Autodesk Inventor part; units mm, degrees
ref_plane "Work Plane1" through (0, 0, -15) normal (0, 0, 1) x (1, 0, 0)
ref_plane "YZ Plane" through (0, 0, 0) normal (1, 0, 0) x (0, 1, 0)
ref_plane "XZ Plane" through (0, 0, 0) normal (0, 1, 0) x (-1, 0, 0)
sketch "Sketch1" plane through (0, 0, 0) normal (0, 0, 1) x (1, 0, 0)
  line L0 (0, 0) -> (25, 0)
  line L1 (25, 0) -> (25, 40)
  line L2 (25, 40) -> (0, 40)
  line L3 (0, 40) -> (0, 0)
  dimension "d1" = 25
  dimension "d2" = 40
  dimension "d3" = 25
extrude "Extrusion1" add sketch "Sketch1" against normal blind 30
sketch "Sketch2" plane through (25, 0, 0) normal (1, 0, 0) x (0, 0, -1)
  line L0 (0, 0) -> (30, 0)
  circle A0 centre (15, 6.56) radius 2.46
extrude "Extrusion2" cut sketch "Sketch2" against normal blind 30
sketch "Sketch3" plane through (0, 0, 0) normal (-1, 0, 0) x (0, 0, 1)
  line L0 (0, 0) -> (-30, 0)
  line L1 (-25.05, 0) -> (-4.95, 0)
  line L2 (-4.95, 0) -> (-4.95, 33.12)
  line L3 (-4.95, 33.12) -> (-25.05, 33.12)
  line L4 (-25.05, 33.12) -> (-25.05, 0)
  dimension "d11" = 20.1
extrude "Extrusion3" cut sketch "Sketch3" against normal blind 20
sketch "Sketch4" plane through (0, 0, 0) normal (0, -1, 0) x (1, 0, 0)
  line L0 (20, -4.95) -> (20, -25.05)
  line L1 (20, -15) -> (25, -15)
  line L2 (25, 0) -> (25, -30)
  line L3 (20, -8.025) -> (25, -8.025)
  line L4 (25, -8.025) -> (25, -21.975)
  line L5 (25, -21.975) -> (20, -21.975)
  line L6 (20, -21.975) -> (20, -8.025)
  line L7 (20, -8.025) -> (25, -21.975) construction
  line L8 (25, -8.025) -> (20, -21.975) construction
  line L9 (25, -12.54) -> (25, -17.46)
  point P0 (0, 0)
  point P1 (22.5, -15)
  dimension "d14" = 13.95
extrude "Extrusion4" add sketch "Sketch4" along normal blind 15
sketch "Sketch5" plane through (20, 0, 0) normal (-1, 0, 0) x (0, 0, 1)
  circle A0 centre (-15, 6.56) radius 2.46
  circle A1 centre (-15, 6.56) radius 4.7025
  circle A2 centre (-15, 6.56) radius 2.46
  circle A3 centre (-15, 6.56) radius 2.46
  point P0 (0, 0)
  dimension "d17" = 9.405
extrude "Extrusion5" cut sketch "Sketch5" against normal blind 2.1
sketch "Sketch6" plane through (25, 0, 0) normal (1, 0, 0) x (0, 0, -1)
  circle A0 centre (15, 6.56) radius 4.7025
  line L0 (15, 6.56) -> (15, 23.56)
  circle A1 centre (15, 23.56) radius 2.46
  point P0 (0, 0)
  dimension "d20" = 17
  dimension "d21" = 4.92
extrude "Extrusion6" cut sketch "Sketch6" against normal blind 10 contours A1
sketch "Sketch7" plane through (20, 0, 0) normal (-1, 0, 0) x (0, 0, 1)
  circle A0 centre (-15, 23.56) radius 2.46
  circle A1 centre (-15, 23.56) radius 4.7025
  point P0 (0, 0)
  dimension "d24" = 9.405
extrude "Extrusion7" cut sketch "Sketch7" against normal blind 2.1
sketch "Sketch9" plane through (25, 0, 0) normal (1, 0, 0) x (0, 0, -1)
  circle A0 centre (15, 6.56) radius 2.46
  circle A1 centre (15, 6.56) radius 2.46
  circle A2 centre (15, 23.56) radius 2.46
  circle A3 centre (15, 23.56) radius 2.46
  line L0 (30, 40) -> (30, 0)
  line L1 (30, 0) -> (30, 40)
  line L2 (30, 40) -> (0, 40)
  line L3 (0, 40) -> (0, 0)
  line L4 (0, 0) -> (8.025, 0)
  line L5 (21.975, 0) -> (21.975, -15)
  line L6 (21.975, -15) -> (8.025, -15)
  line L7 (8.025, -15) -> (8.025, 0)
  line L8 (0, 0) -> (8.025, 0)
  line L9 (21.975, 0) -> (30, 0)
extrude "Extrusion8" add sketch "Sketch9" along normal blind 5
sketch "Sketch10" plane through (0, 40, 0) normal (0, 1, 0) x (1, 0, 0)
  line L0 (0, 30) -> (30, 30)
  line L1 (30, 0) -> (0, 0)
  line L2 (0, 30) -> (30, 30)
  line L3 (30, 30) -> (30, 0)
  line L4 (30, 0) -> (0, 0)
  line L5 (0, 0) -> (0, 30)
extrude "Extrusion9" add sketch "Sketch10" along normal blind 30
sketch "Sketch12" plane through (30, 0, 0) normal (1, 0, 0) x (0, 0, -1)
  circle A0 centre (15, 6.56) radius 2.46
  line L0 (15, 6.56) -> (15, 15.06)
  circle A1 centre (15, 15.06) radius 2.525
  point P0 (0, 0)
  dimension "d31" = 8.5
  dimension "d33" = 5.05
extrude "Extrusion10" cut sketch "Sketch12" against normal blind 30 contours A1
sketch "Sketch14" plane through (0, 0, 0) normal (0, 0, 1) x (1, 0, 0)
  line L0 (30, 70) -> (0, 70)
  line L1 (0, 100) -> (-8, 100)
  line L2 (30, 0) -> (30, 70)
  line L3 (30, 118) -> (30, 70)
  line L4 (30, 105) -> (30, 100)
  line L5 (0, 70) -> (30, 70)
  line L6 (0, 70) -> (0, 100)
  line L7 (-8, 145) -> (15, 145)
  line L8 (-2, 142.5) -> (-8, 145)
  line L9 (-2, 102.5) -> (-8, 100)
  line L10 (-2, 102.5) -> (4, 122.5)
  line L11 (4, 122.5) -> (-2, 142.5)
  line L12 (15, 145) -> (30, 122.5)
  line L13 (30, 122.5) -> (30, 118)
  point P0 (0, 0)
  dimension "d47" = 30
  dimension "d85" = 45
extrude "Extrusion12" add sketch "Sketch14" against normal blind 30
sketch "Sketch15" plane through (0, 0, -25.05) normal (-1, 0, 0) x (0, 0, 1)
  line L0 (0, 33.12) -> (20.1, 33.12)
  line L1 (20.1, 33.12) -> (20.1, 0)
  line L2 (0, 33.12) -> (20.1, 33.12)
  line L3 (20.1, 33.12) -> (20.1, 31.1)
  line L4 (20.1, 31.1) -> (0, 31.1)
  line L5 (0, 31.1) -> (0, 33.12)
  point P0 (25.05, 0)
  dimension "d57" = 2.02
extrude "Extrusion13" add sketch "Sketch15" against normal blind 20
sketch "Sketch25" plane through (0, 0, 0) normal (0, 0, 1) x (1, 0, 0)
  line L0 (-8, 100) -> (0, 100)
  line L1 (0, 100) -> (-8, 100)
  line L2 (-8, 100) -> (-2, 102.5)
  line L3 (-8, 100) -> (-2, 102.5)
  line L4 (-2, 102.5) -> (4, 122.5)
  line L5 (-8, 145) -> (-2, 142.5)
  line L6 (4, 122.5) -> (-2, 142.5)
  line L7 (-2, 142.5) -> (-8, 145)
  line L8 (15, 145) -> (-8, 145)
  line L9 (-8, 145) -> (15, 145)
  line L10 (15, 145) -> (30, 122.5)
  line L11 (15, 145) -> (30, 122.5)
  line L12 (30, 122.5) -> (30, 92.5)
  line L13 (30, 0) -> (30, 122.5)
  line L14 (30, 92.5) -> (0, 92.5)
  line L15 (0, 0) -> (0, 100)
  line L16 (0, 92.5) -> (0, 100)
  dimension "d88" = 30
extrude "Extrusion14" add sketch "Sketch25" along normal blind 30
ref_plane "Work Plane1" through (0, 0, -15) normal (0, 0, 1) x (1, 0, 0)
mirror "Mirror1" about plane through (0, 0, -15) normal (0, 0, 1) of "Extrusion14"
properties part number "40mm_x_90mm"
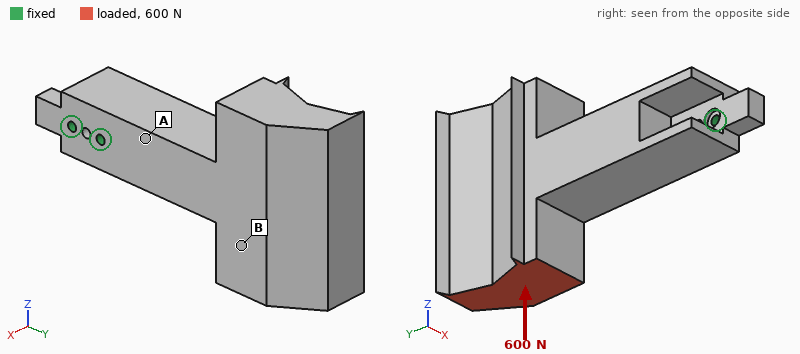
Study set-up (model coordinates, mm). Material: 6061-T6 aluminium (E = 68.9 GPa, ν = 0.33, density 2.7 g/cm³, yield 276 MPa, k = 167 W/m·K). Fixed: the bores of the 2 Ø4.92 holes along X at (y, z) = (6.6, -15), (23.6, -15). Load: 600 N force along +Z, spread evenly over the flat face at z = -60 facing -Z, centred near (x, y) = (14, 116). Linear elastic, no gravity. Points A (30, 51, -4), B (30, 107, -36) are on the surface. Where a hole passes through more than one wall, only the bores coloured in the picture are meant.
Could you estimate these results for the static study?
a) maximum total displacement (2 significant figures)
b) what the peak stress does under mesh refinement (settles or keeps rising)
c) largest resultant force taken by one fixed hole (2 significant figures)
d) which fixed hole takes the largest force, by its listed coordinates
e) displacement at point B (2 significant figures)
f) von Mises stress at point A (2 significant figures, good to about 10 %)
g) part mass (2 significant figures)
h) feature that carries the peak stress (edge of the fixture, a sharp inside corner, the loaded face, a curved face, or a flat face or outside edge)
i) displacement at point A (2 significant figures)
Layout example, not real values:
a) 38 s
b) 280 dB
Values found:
a) 0.16 mm
b) keeps rising
c) 3.0 kN
d) (23.6, -15)
e) 0.099 mm
f) 8.0 MPa
g) 530 g
h) edge of the fixture
i) 0.027 mm
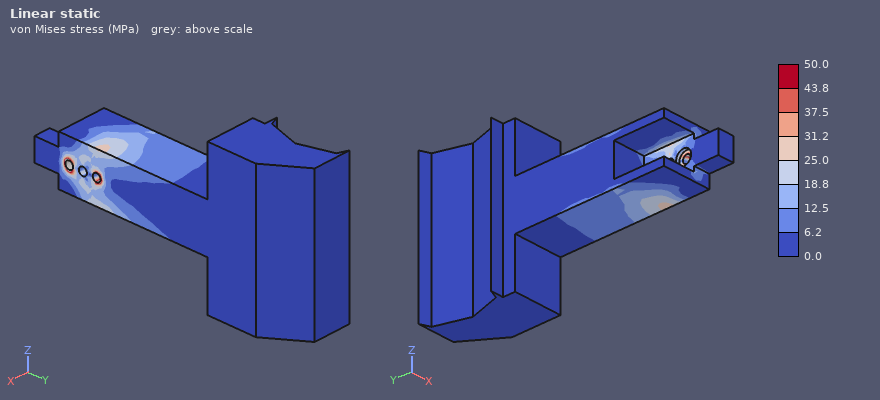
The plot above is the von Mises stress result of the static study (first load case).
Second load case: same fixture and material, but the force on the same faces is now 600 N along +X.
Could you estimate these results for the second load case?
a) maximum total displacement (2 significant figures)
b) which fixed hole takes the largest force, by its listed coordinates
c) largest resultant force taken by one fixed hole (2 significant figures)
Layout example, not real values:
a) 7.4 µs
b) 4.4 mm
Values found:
a) 0.29 mm
b) (23.6, -15)
c) 2.8 kN
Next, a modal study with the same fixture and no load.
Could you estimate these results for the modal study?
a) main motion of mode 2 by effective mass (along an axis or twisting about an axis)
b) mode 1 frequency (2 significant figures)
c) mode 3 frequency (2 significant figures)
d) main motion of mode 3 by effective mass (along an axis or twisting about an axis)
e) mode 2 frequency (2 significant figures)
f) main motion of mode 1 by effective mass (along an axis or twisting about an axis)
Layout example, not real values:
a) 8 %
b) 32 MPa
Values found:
a) along Z
b) 520 Hz
c) 1200 Hz
d) twisting about Y
e) 590 Hz
f) along X
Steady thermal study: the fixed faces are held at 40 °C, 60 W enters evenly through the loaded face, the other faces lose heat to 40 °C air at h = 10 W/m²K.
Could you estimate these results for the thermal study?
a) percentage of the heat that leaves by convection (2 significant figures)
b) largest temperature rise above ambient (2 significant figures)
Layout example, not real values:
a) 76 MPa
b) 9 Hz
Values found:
a) 14 %
b) 48 K
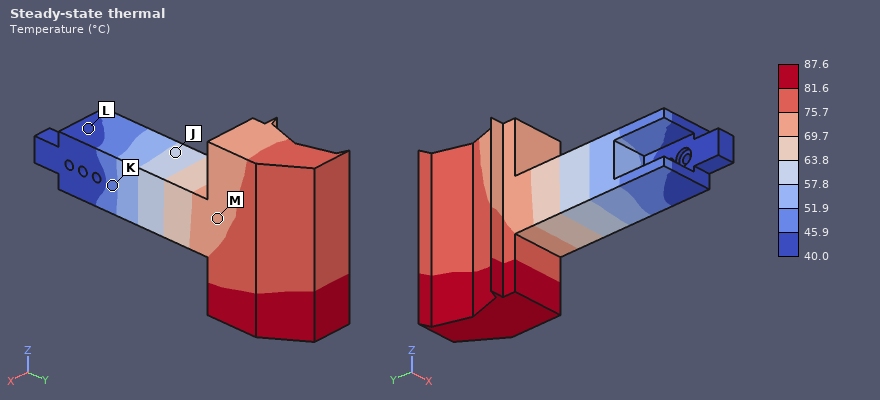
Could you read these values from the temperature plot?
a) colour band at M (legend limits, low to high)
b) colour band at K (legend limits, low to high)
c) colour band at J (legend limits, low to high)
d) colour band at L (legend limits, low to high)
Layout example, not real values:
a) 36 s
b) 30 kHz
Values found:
a) 69.7 to 75.7 °C
b) 45.9 to 51.9 °C
c) 57.8 to 63.8 °C
d) 40.0 to 45.9 °C
